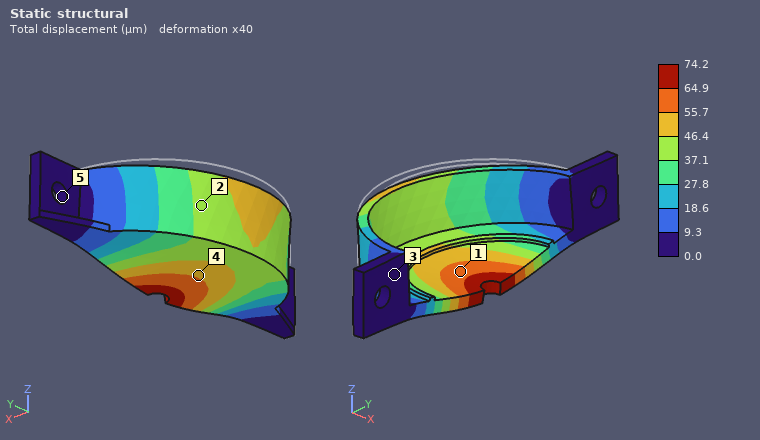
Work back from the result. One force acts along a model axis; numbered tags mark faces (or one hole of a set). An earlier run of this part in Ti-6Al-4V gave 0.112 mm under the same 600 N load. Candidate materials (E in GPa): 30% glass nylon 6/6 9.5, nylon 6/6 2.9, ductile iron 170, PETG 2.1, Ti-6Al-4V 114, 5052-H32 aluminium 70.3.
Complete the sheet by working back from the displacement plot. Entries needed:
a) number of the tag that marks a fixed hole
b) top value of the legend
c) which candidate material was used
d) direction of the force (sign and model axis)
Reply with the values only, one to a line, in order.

5
74.2 µm
ductile iron
-Z
